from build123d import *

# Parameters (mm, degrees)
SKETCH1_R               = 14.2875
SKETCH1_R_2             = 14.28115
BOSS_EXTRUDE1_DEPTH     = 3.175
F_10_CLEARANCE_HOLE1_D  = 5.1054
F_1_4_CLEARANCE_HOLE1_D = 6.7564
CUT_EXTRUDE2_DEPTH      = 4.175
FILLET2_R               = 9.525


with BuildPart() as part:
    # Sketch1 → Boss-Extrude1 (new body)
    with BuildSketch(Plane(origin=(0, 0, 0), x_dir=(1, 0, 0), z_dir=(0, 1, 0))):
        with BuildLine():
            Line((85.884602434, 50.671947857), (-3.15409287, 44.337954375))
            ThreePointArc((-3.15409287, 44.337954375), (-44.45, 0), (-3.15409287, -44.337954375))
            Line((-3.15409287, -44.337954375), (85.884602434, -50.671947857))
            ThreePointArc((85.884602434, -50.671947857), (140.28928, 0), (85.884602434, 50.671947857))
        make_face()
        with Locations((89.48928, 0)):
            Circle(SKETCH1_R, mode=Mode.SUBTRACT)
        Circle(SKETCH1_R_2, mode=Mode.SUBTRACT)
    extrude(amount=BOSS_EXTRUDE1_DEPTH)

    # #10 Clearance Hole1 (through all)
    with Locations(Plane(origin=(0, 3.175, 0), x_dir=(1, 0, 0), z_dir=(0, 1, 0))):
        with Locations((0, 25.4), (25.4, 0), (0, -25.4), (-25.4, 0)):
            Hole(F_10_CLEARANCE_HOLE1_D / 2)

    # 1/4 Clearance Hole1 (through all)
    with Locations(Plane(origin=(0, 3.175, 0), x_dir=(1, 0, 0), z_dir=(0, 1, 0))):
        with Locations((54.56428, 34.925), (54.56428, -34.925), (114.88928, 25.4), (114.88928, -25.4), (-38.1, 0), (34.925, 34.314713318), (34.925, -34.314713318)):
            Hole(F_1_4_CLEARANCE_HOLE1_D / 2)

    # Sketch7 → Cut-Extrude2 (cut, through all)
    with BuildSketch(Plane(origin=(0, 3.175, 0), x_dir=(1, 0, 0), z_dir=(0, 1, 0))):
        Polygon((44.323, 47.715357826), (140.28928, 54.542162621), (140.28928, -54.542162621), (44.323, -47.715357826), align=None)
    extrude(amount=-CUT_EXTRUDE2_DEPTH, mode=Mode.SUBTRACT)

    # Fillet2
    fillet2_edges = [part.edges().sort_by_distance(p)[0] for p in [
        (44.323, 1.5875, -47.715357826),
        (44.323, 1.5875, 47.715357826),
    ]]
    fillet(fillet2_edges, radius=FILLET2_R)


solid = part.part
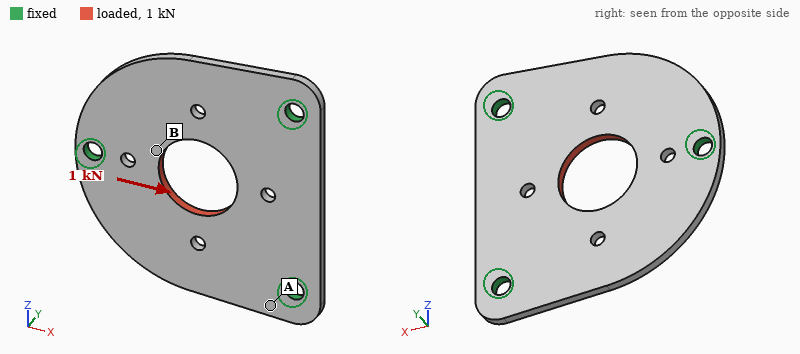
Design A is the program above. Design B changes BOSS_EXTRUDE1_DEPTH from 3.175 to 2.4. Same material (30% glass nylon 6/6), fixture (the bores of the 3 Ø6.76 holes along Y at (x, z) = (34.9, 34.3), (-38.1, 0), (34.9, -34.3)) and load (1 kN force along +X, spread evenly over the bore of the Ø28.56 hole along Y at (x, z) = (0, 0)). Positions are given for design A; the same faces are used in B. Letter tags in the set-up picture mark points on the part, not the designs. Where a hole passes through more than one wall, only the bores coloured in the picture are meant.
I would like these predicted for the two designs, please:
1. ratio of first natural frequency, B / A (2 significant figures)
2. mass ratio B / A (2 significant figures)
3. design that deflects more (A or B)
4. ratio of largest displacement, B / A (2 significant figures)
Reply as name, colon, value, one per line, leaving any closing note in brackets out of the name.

ratio of first natural frequency, B / A: 0.77
mass ratio B / A: 0.76
design that deflects more: B
ratio of largest displacement, B / A: 1.3
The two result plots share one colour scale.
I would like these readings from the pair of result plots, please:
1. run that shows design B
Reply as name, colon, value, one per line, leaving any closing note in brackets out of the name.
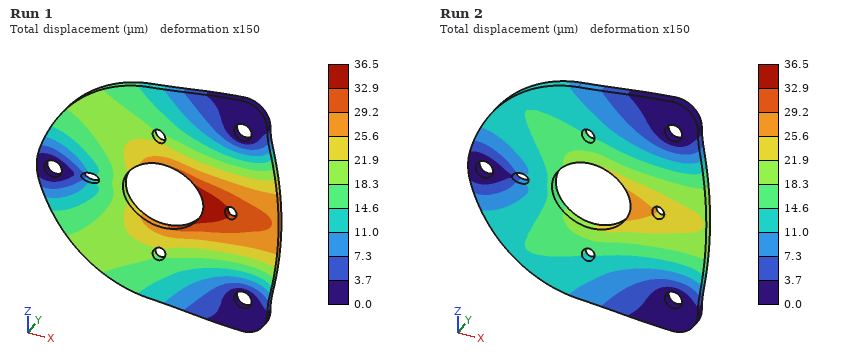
run that shows design B: Run 1
